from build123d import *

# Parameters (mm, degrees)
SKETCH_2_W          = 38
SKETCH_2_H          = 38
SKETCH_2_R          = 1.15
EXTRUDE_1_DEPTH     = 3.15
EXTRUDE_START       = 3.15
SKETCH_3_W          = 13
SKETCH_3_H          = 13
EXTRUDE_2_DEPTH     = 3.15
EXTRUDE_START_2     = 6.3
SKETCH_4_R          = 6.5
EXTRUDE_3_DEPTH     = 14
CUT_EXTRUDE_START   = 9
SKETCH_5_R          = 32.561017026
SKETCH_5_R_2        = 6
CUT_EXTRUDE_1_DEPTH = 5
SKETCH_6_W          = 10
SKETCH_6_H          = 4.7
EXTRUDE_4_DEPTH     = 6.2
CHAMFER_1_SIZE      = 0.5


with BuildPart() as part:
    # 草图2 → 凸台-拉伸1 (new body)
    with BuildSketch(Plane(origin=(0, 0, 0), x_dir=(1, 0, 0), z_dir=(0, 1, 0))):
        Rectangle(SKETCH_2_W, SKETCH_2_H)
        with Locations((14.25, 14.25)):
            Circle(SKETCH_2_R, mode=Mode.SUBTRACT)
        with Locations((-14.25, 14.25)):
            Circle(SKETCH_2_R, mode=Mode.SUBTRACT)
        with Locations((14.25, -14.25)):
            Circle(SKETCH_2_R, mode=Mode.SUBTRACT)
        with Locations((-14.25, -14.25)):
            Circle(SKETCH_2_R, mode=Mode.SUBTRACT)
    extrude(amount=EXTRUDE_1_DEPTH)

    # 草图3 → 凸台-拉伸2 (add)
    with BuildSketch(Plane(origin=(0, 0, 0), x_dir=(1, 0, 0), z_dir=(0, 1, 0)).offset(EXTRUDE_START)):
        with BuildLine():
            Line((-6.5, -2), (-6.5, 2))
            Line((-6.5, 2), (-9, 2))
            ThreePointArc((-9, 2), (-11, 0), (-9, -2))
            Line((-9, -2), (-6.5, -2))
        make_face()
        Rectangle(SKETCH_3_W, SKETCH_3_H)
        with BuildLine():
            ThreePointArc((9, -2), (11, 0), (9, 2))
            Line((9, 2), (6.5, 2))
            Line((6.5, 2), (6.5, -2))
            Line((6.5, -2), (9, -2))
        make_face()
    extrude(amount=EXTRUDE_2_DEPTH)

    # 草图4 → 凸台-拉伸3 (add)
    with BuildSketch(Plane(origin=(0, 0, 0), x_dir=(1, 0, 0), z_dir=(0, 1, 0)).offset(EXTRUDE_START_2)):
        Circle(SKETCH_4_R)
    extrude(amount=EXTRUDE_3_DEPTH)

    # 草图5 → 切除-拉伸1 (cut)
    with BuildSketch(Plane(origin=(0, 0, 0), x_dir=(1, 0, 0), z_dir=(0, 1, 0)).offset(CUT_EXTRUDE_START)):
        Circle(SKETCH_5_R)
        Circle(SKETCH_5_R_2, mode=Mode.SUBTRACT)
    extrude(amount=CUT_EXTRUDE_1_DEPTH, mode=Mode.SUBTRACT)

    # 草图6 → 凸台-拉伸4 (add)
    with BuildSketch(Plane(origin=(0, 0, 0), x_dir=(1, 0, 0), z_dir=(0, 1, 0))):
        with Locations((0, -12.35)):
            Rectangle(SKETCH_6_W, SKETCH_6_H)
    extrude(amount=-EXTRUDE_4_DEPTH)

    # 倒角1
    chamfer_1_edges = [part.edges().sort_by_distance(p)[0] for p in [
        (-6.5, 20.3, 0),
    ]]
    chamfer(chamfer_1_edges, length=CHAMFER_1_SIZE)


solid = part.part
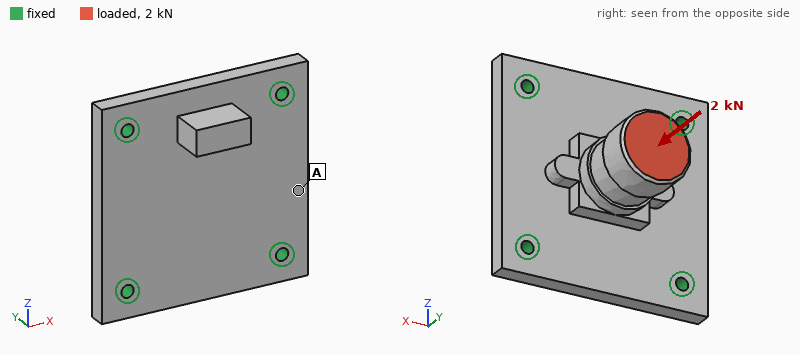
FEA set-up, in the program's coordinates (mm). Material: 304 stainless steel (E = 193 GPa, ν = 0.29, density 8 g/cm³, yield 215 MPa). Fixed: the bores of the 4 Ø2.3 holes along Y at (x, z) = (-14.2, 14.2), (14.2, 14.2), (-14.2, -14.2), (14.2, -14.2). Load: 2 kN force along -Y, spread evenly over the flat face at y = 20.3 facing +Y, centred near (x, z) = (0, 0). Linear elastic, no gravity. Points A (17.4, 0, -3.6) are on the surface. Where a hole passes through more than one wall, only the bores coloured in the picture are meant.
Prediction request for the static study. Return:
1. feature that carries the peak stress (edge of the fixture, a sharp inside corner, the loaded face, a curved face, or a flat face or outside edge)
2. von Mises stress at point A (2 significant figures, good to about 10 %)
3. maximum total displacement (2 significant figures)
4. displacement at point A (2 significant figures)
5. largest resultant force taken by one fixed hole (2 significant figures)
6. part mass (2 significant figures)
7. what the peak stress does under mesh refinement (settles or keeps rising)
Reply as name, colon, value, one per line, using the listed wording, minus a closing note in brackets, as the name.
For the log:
feature that carries the peak stress: edge of the fixture
von Mises stress at point A: 44 MPa
maximum total displacement: 19 µm
displacement at point A: 7.3 µm
largest resultant force taken by one fixed hole: 520 N
part mass: 57 g
what the peak stress does under mesh refinement: keeps rising
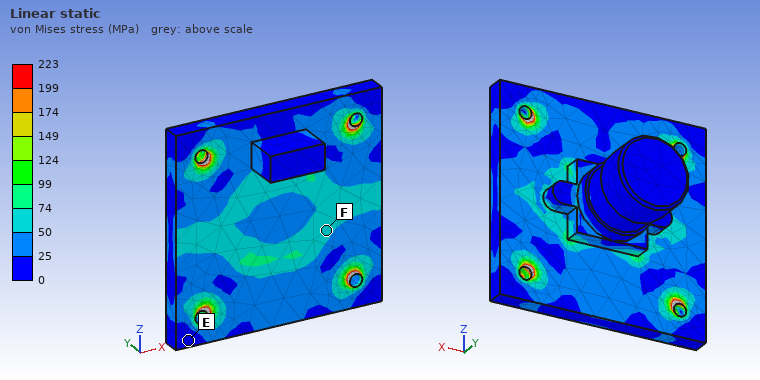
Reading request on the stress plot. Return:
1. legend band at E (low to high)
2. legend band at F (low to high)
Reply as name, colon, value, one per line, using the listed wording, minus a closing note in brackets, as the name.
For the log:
legend band at E: 0 to 25 MPa
legend band at F: 50 to 74 MPa
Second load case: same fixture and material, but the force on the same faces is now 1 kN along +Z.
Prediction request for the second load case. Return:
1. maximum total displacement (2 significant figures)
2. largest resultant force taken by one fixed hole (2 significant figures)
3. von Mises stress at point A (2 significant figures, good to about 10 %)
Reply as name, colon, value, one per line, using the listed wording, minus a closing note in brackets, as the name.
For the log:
maximum total displacement: 37 µm
largest resultant force taken by one fixed hole: 480 N
von Mises stress at point A: 21 MPa
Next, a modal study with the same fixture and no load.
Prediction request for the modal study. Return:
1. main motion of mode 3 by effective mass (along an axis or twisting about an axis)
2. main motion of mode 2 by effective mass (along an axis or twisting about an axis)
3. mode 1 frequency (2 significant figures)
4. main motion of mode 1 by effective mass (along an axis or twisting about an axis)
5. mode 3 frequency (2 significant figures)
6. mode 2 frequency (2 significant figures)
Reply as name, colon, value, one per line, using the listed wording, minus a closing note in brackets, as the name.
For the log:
main motion of mode 3 by effective mass: along X
main motion of mode 2 by effective mass: along Z
mode 1 frequency: 9400 Hz
main motion of mode 1 by effective mass: along Y
mode 3 frequency: 10 kHz
mode 2 frequency: 9900 Hz
